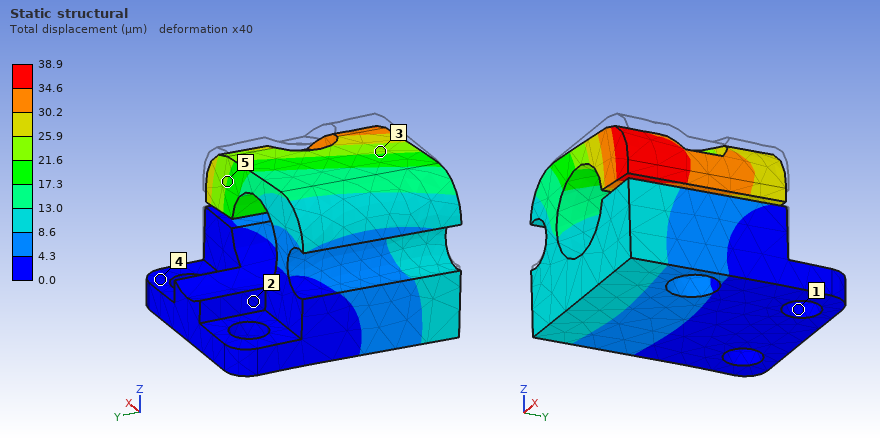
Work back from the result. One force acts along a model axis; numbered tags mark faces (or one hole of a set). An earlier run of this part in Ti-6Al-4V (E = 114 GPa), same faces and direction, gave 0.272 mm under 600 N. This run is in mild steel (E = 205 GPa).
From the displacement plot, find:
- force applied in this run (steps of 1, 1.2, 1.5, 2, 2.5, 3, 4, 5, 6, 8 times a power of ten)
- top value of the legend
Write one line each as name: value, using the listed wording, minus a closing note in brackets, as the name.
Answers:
force applied in this run: 150 N
top value of the legend: 38.9 µm
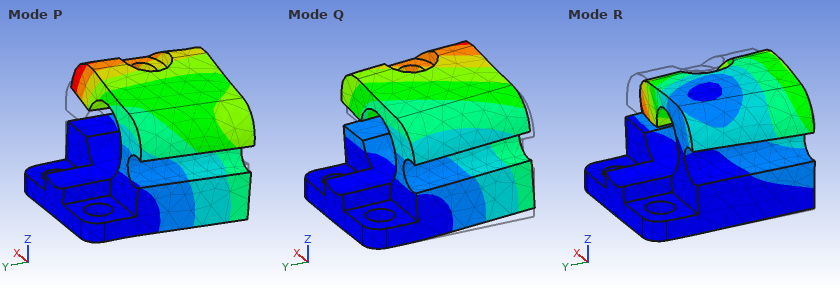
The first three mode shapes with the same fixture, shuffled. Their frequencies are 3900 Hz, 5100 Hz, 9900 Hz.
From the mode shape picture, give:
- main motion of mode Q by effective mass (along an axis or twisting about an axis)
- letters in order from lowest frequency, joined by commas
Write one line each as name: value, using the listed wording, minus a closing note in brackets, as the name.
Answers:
main motion of mode Q by effective mass: along Z
letters in order from lowest frequency, joined by commas: Q, P, R
